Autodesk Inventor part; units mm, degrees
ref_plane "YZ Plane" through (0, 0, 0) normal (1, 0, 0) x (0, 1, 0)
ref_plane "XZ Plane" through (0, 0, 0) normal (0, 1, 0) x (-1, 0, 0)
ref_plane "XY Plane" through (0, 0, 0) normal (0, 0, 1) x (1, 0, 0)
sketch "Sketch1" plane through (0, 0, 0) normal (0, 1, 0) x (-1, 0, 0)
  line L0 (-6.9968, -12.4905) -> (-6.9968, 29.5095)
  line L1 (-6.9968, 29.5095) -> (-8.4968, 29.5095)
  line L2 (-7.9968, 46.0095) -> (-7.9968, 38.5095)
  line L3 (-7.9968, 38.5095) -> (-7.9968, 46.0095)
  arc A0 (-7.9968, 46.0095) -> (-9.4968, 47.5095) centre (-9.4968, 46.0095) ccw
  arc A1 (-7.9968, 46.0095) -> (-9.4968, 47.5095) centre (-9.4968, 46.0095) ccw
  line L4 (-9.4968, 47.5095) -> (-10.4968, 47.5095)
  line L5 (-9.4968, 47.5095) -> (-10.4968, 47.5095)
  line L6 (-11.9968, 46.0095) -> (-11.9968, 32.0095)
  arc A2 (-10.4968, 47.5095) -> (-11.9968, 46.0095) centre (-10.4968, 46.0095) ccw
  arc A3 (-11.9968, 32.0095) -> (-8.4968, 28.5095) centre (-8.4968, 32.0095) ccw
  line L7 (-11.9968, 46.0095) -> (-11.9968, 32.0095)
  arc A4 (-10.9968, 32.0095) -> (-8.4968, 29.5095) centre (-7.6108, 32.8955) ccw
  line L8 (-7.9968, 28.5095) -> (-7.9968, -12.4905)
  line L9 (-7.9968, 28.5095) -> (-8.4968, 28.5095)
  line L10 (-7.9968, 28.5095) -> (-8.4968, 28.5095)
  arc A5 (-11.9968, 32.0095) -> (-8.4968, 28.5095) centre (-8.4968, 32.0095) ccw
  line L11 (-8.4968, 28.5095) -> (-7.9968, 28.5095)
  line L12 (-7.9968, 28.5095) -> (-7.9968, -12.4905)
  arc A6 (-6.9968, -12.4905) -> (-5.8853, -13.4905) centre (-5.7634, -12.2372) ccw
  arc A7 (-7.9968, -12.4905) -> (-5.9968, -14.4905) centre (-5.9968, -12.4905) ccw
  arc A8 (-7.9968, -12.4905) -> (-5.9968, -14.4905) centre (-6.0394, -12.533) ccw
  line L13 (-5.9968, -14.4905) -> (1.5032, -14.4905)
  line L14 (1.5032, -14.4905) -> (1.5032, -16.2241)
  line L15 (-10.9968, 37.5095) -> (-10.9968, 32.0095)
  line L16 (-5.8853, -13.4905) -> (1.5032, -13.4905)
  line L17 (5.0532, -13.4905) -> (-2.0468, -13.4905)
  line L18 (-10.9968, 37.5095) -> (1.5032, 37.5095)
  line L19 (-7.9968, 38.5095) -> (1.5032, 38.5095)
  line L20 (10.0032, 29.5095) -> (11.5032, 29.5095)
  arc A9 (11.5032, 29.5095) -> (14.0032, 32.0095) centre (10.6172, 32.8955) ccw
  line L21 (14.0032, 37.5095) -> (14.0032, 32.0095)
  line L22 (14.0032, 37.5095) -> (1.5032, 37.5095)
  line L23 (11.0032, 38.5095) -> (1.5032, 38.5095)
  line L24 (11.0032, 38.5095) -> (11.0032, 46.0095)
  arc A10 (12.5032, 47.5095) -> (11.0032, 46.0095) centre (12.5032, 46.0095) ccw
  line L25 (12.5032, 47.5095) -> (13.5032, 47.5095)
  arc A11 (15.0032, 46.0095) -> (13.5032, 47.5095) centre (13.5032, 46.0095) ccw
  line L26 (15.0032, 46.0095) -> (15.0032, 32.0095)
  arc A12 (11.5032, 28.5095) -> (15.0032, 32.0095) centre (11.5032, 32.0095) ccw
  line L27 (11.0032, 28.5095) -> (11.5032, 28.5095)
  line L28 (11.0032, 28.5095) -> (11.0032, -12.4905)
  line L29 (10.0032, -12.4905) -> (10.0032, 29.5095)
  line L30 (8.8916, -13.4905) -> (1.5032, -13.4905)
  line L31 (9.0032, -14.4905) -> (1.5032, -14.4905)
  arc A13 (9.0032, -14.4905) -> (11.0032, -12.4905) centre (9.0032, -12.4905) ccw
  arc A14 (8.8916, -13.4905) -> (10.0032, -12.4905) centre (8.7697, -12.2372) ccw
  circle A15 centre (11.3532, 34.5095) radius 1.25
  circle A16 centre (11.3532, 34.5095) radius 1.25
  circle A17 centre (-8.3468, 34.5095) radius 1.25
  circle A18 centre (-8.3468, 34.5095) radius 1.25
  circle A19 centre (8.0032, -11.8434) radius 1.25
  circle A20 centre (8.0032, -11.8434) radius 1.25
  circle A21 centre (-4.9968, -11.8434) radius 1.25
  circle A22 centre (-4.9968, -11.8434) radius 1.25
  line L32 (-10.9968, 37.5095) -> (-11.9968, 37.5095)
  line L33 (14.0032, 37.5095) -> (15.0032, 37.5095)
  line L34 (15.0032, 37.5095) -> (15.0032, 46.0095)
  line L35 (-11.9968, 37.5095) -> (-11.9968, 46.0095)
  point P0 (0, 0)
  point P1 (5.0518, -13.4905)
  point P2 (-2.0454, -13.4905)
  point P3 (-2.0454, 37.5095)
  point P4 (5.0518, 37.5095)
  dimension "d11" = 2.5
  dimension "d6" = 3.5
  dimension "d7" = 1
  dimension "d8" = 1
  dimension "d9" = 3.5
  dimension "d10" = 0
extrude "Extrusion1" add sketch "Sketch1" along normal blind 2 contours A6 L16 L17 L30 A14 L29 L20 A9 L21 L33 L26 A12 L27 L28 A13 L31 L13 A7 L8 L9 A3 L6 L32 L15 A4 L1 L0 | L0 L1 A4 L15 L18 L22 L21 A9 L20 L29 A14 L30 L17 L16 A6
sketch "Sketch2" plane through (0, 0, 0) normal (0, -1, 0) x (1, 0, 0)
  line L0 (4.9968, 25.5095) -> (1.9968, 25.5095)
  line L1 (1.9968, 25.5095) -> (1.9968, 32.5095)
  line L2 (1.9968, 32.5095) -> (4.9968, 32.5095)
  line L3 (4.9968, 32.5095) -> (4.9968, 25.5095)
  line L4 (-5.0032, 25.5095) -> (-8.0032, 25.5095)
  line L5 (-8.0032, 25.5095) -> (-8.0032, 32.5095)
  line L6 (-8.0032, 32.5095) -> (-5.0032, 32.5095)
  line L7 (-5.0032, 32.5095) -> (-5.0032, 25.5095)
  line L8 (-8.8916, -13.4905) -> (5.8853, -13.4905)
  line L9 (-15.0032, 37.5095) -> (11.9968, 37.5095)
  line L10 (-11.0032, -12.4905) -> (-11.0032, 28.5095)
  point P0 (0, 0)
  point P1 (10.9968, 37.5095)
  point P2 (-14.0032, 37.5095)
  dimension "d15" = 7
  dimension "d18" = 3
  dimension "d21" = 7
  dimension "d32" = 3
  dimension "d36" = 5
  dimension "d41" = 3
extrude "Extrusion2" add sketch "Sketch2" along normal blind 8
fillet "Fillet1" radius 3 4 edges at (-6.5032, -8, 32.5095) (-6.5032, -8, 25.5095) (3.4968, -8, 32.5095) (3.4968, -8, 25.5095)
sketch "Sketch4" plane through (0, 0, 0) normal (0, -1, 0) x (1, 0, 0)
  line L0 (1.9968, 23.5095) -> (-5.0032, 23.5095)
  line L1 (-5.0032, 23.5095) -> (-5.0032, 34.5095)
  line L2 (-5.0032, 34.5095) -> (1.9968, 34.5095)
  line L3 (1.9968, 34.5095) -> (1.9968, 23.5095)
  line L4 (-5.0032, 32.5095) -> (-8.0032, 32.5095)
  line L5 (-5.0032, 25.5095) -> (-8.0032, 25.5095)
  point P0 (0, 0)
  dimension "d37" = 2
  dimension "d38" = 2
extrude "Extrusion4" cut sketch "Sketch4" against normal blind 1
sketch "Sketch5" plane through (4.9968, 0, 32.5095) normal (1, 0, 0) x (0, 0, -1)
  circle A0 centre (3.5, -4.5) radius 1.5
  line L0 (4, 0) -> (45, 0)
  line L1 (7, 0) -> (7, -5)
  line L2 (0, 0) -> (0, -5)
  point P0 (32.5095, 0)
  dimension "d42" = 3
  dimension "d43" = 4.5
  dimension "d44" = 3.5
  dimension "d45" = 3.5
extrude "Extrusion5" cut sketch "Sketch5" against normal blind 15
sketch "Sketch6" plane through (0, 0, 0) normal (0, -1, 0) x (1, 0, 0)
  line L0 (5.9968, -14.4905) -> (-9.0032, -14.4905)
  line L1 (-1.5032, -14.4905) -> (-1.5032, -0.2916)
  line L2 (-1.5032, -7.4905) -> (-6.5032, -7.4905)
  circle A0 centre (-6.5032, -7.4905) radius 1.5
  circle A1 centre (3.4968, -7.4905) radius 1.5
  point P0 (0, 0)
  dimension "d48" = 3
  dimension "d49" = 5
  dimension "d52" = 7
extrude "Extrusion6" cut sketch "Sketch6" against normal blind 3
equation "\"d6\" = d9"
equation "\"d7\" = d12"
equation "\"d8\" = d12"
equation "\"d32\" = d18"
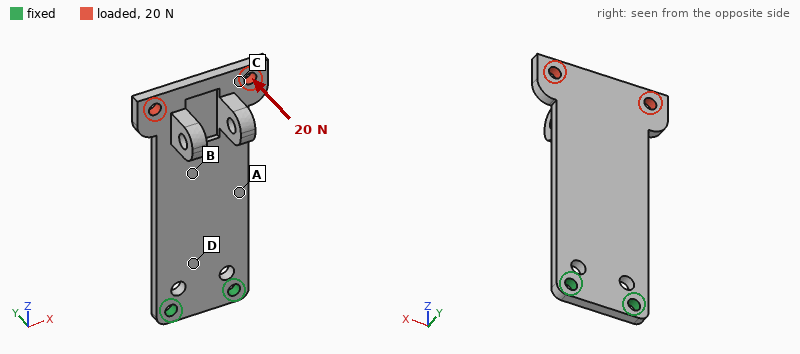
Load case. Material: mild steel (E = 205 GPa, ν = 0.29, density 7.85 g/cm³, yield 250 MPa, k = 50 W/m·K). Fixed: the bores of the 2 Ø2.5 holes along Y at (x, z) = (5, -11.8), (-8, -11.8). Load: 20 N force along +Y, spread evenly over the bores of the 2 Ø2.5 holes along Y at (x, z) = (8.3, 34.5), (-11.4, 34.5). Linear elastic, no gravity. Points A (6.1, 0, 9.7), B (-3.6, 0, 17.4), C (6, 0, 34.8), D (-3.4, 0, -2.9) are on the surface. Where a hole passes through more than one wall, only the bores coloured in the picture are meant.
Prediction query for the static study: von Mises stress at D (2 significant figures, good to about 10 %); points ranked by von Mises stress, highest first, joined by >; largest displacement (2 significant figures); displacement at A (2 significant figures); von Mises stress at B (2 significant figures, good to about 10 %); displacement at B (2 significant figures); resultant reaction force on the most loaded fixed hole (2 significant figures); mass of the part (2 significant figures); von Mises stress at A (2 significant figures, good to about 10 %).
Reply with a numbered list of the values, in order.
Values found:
1. 58 MPa
2. D > A > B > C
3. 0.31 mm
4. 0.079 mm
5. 25 MPa
6. 0.13 mm
7. 10 N
8. 18 g
9. 39 MPa
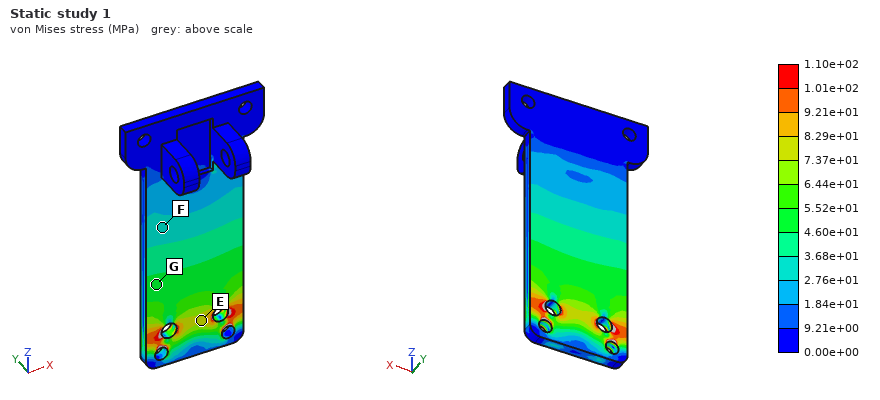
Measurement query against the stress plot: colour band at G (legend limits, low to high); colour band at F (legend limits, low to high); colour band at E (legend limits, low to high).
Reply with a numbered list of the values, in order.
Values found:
1. 4.60e+01 to 5.52e+01 MPa
2. 2.76e+01 to 3.68e+01 MPa
3. 7.37e+01 to 8.29e+01 MPa
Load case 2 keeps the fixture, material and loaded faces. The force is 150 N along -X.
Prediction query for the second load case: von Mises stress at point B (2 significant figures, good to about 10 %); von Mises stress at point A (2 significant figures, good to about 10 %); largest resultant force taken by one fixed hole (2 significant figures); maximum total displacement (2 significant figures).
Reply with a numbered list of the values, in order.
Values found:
1. 12 MPa
2. 25 MPa
3. 480 N
4. 32 µm
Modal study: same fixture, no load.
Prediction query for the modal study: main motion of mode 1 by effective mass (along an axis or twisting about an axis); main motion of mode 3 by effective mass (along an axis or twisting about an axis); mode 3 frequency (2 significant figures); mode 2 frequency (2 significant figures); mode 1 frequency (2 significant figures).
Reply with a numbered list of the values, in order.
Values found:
1. along Y
2. along Y
3. 3800 Hz
4. 2400 Hz
5. 540 Hz
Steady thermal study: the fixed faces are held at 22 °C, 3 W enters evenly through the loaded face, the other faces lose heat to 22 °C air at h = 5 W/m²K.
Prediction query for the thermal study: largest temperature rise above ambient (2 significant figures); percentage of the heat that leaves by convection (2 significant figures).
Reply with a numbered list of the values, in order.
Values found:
1. 72 K
2. 18 %
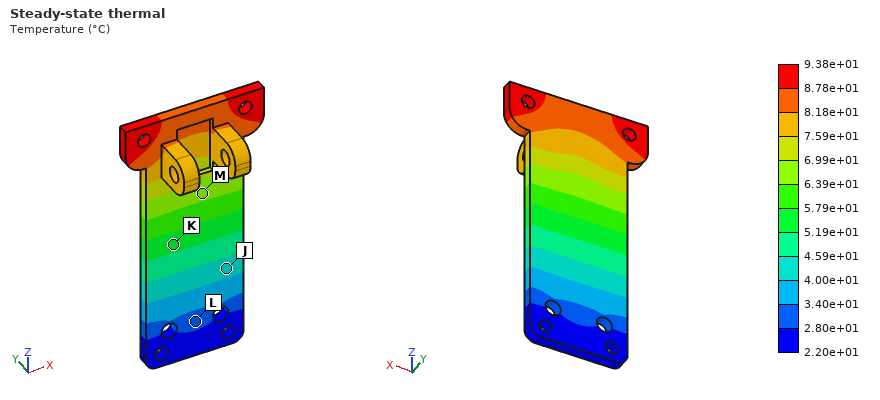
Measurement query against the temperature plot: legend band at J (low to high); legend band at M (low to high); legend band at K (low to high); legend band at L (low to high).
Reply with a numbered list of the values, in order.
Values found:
1. 4.00e+01 to 4.59e+01 °C
2. 6.39e+01 to 6.99e+01 °C
3. 5.19e+01 to 5.79e+01 °C
4. 2.80e+01 to 3.40e+01 °C
